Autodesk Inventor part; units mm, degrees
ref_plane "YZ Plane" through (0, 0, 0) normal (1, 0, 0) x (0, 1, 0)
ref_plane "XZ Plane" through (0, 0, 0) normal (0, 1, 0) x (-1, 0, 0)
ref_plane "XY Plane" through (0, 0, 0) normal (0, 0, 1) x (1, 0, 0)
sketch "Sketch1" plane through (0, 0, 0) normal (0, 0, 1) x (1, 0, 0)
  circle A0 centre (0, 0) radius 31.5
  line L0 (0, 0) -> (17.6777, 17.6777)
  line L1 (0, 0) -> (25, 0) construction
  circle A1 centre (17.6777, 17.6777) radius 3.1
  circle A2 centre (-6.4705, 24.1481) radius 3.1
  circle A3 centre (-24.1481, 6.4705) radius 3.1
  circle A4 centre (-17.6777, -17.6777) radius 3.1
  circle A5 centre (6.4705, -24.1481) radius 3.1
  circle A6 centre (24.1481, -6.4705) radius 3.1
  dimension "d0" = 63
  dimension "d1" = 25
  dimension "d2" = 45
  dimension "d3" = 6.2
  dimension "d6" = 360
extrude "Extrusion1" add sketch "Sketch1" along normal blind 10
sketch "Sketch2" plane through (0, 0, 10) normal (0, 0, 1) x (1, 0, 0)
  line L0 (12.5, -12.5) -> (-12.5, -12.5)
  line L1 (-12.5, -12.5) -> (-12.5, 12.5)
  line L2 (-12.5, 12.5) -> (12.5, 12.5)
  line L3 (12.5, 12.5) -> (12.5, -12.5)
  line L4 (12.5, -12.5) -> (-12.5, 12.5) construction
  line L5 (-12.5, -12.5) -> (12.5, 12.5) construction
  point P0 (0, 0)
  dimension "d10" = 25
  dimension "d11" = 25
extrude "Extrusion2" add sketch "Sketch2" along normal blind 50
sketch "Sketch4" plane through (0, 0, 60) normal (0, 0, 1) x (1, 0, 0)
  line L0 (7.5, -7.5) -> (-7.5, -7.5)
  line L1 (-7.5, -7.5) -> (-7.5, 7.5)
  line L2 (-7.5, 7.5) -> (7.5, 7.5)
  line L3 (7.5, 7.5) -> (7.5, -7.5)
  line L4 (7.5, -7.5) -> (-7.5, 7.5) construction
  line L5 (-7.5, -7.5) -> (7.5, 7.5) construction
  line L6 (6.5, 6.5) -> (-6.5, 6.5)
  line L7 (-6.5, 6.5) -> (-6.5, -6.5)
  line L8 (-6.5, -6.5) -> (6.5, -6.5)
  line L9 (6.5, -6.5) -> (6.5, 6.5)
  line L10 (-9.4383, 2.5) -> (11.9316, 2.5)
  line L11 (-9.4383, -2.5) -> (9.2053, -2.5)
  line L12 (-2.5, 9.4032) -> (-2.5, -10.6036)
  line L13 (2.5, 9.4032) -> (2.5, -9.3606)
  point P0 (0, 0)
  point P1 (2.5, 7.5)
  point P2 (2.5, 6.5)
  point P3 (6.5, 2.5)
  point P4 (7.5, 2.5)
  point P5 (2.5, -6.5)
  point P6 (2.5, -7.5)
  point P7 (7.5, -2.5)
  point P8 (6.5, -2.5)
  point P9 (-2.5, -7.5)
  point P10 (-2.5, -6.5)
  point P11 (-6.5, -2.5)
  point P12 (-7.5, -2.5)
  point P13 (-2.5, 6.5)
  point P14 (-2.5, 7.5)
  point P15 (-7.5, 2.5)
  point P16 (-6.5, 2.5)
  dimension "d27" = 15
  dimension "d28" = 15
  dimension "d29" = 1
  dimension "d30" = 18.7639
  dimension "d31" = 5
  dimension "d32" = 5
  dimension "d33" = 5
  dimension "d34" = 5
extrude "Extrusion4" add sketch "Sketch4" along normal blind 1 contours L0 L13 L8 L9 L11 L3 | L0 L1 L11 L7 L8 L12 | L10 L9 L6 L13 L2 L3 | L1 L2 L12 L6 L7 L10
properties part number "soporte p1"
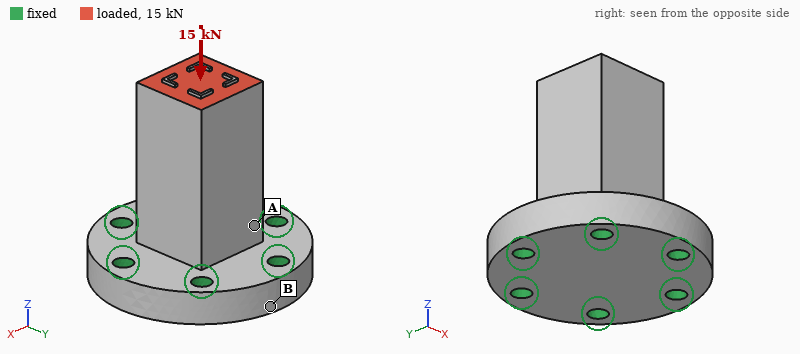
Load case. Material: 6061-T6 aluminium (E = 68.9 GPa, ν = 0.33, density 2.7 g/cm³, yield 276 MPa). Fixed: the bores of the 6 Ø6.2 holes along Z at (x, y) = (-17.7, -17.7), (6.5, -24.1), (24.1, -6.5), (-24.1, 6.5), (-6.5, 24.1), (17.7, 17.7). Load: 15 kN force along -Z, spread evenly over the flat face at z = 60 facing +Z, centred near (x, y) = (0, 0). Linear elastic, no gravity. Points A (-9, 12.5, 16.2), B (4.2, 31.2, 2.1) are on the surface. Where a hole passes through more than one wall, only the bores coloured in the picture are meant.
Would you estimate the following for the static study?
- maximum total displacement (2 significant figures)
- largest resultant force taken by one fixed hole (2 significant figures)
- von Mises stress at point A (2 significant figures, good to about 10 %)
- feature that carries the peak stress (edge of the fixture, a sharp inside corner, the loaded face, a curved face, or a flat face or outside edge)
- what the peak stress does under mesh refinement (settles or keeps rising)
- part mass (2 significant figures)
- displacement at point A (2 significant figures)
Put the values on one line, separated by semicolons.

31 µm; 2.8 kN; 32 MPa; edge of the fixture; keeps rising; 160 g; 15 µm
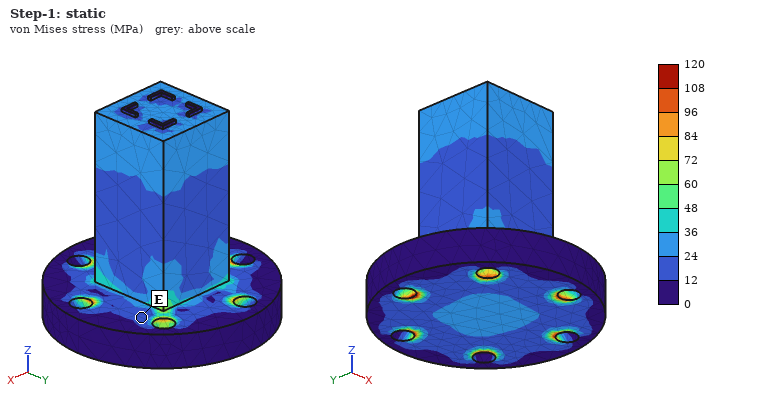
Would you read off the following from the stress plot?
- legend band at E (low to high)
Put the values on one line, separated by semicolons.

12 to 24 MPa
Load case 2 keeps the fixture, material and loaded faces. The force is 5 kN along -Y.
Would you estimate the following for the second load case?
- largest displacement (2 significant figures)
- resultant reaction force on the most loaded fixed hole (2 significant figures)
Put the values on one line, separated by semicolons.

0.18 mm; 4.1 kN
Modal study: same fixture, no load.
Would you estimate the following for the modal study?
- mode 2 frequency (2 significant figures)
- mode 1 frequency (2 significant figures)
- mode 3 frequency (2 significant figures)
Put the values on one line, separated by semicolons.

5200 Hz; 5200 Hz; 13 kHz
